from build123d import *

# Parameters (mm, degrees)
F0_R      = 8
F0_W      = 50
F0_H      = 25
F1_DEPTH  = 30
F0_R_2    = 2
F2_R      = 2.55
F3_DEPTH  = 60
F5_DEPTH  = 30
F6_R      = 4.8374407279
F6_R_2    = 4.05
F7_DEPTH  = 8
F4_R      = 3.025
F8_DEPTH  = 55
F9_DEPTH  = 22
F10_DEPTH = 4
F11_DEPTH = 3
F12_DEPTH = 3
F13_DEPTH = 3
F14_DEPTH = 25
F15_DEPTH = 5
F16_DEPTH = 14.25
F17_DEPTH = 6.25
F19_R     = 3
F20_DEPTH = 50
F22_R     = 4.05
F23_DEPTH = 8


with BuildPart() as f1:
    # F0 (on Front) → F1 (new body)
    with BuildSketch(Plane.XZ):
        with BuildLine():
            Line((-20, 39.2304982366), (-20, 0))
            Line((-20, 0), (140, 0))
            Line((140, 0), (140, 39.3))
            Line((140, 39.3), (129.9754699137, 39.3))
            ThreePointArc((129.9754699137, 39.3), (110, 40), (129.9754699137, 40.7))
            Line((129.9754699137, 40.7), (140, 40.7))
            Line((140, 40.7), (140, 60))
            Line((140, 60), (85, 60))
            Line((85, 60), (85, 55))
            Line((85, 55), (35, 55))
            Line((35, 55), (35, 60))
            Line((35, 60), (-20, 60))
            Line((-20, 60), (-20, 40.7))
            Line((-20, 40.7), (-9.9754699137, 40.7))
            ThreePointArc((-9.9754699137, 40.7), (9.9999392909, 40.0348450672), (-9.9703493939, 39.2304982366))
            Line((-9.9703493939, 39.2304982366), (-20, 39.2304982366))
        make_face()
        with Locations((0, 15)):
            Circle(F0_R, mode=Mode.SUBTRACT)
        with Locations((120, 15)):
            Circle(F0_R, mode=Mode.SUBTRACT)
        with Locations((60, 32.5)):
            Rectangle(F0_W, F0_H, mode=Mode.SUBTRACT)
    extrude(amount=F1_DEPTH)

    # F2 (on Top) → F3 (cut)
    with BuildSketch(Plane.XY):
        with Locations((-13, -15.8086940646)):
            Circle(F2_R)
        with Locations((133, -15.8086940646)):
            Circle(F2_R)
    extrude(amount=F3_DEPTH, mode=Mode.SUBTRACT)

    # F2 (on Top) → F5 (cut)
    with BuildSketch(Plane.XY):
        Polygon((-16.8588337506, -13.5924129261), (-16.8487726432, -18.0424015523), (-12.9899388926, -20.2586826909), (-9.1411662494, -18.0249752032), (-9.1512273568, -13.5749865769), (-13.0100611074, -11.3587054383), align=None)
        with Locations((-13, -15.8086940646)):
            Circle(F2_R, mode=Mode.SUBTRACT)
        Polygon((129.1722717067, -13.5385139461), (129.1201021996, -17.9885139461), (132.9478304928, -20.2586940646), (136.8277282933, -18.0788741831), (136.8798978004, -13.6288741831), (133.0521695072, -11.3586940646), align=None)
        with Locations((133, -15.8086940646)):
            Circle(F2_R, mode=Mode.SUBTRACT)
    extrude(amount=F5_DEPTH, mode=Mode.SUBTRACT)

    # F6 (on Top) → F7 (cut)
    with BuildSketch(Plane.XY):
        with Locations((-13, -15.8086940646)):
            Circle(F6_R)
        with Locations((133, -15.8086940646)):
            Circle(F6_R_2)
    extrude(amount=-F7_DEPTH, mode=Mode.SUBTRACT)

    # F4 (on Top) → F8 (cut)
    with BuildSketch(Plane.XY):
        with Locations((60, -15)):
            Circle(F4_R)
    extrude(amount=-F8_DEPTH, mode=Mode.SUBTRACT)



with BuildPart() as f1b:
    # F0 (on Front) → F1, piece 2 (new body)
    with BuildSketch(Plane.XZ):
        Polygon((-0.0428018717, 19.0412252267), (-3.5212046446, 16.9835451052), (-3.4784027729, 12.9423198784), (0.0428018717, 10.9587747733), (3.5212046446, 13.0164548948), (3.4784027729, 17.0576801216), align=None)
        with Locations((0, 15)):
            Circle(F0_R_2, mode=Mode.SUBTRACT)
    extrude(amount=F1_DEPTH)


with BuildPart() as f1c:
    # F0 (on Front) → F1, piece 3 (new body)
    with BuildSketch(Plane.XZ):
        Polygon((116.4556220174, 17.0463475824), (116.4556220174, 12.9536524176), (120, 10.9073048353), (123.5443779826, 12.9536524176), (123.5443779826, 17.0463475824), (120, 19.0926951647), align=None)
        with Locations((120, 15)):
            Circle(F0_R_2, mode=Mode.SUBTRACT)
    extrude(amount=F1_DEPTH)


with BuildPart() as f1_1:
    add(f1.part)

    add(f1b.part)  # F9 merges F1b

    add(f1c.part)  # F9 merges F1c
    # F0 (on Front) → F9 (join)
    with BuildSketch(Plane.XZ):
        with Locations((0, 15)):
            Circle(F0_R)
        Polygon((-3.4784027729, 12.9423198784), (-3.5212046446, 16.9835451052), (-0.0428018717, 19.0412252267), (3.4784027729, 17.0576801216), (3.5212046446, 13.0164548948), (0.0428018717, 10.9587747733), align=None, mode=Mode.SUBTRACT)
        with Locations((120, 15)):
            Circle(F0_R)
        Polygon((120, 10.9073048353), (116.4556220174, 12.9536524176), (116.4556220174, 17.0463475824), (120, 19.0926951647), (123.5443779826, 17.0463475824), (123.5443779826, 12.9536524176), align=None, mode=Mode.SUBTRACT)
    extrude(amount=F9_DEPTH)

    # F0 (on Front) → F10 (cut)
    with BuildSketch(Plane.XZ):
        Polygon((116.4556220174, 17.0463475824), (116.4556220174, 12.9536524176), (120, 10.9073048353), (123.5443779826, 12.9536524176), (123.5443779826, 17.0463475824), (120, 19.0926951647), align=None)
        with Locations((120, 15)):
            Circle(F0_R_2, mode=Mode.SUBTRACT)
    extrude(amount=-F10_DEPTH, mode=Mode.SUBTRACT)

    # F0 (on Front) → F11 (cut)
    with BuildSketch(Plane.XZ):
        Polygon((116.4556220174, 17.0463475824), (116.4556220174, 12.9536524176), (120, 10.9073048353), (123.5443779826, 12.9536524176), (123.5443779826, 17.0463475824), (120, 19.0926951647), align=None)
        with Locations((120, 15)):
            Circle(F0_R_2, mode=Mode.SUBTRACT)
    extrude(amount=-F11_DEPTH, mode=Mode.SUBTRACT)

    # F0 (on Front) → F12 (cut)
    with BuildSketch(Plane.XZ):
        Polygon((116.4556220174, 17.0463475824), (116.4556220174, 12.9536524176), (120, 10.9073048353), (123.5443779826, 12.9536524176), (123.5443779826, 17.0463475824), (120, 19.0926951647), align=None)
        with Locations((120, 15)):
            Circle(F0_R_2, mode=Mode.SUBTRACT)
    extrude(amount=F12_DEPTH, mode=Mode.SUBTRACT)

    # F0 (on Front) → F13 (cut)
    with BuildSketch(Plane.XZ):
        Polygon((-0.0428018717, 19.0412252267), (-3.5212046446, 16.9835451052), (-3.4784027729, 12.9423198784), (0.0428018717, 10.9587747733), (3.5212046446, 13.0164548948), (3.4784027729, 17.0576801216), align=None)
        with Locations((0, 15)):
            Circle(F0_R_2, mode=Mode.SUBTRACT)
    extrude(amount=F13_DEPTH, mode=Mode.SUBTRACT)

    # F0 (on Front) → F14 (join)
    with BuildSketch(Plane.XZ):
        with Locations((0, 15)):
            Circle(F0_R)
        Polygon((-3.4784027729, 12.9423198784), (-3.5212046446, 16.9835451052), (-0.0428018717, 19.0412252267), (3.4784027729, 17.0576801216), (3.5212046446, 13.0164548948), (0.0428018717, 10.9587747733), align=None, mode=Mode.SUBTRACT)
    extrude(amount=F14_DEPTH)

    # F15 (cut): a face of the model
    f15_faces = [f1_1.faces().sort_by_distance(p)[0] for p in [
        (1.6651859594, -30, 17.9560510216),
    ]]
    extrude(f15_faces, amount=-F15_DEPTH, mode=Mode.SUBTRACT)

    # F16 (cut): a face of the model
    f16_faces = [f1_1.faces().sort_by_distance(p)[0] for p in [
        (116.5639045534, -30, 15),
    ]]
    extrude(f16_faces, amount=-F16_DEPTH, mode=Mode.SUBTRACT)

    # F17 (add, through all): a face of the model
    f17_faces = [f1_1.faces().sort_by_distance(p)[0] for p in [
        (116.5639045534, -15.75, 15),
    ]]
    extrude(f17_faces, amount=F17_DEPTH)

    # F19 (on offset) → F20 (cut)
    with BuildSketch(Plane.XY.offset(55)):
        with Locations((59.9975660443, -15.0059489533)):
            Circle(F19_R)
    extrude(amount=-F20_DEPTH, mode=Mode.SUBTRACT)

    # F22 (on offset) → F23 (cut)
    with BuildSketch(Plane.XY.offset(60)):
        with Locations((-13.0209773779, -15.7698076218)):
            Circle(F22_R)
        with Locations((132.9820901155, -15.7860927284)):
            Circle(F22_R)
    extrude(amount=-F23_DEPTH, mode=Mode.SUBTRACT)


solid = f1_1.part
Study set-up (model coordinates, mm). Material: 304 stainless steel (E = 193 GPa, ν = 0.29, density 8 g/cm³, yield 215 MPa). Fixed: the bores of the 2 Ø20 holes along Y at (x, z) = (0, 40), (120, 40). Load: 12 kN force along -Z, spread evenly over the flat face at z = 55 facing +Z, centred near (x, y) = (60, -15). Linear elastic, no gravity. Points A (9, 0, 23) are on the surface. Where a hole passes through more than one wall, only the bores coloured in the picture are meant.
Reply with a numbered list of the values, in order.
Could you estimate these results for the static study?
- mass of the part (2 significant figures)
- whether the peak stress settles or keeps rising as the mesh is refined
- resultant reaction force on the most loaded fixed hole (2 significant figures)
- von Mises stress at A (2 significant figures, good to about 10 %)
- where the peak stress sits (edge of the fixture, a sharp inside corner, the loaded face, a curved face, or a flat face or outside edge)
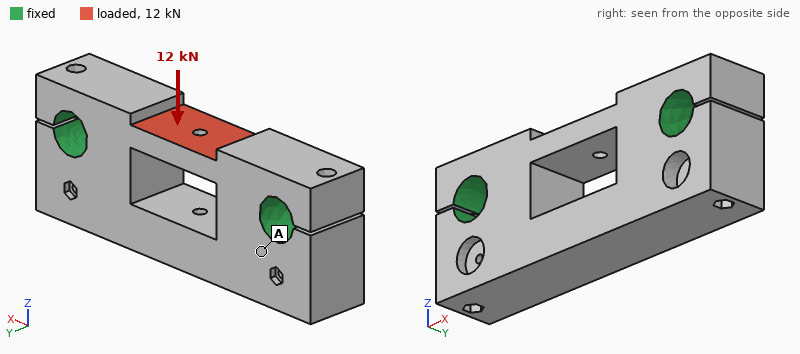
1. 1.7 kg
2. keeps rising
3. 6.1 kN
4. 8.5 MPa
5. a sharp inside corner
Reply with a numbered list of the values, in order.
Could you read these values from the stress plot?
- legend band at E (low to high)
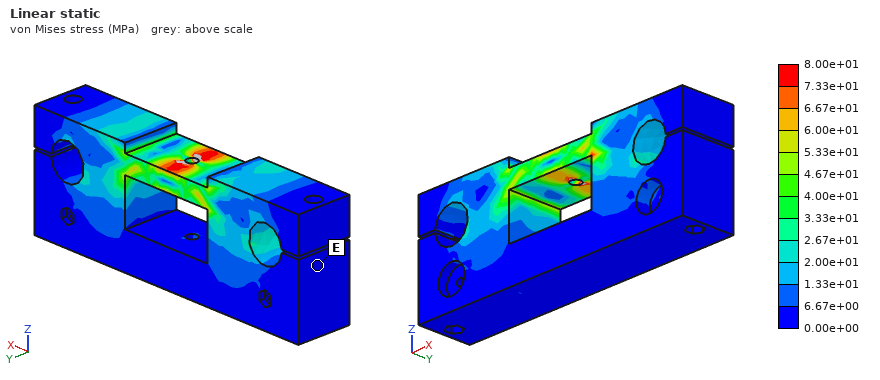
1. 0.00e+00 to 6.67e+00 MPa
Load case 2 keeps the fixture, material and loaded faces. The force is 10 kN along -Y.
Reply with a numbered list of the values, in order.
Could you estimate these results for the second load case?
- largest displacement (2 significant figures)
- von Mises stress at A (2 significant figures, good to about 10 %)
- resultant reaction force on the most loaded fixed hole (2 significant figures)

1. 17 µm
2. 7.8 MPa
3. 5.0 kN
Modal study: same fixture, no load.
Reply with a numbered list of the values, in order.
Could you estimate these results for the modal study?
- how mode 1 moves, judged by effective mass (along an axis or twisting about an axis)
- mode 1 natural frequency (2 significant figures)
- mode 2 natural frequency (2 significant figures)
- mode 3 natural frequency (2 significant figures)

1. along Y
2. 7600 Hz
3. 10 kHz
4. 11 kHz
